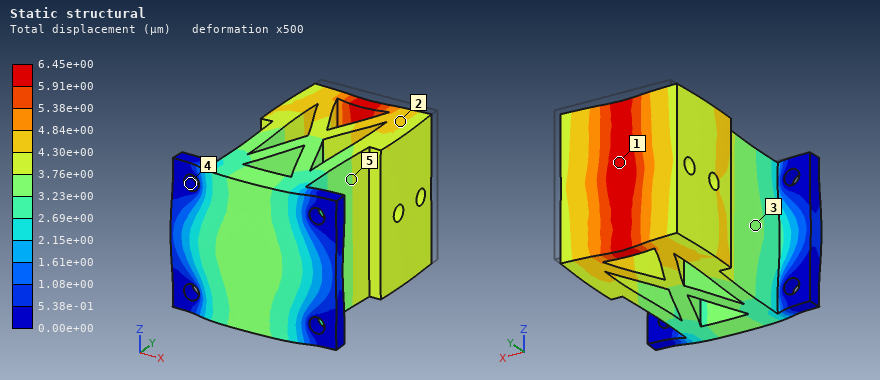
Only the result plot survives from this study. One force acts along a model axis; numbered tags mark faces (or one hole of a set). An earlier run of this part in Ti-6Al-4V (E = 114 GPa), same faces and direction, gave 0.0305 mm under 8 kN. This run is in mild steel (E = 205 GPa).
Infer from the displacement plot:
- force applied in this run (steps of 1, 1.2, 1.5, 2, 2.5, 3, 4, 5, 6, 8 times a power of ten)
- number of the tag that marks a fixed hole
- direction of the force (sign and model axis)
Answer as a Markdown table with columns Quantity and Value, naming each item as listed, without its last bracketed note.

| Quantity | Value |
|---|---|
| force applied in this run | 3 kN |
| number of the tag that marks a fixed hole | 4 |
| direction of the force | -Y |
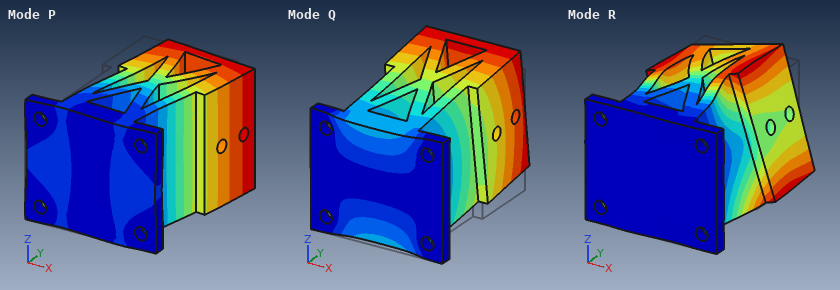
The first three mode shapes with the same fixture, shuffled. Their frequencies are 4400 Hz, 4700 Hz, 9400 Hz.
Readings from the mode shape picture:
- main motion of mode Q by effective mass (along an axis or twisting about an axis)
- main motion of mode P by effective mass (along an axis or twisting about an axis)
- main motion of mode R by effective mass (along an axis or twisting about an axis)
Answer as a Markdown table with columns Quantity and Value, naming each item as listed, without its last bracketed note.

| Quantity | Value |
|---|---|
| main motion of mode Q by effective mass | along Z |
| main motion of mode P by effective mass | along X |
| main motion of mode R by effective mass | twisting about Y |
